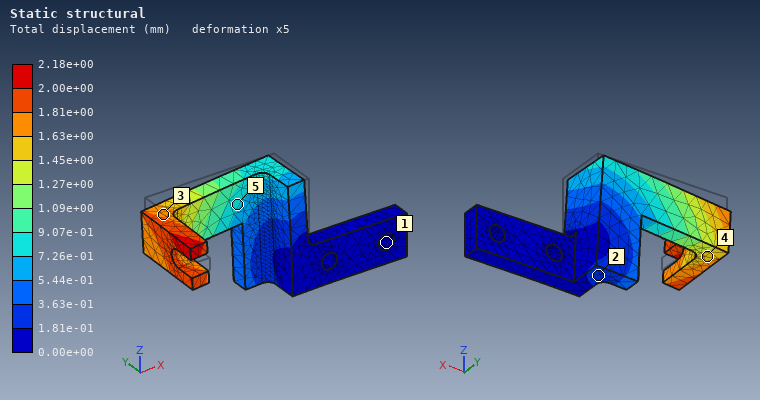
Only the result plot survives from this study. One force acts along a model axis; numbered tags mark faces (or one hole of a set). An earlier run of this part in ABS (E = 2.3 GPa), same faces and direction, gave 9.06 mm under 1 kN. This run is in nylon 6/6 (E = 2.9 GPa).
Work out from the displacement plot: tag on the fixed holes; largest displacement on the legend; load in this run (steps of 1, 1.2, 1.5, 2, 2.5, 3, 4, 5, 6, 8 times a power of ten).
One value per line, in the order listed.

1
2.18e+00 mm
300 N
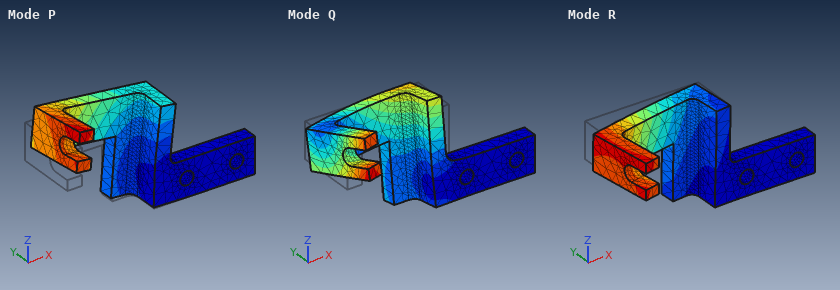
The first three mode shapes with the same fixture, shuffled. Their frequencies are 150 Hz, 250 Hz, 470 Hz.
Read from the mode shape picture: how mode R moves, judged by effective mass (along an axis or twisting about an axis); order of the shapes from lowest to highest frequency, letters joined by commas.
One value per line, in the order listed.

along Y
R, P, Q
